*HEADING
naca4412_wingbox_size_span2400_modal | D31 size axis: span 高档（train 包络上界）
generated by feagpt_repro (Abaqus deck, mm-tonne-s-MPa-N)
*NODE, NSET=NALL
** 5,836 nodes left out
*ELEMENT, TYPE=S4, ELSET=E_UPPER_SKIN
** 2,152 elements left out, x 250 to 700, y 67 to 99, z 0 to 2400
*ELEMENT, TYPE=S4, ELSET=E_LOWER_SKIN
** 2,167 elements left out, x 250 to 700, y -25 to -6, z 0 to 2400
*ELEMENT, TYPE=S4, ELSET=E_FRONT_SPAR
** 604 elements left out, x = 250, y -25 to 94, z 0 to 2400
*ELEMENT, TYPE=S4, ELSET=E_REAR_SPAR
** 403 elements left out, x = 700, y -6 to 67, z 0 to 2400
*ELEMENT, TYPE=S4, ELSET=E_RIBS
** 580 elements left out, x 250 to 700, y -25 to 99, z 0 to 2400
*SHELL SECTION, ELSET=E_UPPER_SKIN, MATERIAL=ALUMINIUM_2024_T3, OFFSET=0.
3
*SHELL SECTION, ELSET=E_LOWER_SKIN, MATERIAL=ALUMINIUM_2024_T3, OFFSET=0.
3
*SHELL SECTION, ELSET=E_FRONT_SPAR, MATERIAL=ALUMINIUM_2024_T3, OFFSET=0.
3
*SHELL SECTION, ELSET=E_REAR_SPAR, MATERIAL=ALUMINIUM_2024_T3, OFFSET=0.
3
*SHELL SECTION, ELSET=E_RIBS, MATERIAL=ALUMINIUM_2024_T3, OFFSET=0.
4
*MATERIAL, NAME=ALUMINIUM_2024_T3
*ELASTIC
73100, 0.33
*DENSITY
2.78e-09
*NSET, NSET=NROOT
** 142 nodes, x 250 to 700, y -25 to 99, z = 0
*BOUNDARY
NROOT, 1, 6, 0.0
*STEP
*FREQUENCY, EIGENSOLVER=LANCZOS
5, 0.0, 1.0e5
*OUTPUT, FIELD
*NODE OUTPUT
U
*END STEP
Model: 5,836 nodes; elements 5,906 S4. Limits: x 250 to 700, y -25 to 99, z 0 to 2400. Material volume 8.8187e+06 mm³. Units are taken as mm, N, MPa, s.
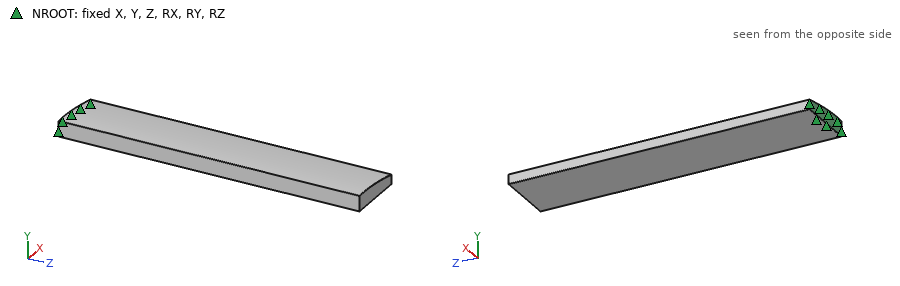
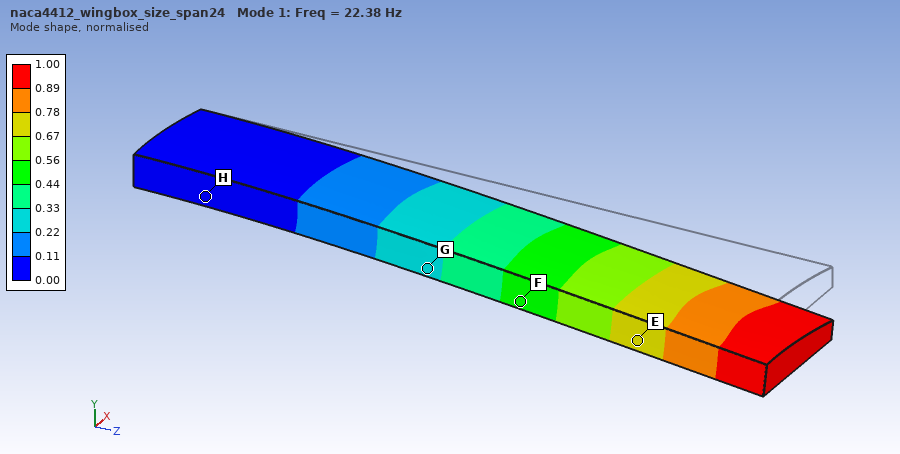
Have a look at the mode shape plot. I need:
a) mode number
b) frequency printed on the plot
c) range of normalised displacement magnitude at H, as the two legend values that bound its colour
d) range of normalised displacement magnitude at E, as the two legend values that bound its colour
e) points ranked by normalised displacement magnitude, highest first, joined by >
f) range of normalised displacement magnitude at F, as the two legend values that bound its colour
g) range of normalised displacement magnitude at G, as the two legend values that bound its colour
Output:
1
22.38 Hz
0.00 to 0.11
0.67 to 0.78
E > F > G > H
0.44 to 0.56
0.22 to 0.33
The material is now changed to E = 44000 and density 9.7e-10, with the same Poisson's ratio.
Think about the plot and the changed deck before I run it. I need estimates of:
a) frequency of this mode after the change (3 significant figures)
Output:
29.4 Hz
